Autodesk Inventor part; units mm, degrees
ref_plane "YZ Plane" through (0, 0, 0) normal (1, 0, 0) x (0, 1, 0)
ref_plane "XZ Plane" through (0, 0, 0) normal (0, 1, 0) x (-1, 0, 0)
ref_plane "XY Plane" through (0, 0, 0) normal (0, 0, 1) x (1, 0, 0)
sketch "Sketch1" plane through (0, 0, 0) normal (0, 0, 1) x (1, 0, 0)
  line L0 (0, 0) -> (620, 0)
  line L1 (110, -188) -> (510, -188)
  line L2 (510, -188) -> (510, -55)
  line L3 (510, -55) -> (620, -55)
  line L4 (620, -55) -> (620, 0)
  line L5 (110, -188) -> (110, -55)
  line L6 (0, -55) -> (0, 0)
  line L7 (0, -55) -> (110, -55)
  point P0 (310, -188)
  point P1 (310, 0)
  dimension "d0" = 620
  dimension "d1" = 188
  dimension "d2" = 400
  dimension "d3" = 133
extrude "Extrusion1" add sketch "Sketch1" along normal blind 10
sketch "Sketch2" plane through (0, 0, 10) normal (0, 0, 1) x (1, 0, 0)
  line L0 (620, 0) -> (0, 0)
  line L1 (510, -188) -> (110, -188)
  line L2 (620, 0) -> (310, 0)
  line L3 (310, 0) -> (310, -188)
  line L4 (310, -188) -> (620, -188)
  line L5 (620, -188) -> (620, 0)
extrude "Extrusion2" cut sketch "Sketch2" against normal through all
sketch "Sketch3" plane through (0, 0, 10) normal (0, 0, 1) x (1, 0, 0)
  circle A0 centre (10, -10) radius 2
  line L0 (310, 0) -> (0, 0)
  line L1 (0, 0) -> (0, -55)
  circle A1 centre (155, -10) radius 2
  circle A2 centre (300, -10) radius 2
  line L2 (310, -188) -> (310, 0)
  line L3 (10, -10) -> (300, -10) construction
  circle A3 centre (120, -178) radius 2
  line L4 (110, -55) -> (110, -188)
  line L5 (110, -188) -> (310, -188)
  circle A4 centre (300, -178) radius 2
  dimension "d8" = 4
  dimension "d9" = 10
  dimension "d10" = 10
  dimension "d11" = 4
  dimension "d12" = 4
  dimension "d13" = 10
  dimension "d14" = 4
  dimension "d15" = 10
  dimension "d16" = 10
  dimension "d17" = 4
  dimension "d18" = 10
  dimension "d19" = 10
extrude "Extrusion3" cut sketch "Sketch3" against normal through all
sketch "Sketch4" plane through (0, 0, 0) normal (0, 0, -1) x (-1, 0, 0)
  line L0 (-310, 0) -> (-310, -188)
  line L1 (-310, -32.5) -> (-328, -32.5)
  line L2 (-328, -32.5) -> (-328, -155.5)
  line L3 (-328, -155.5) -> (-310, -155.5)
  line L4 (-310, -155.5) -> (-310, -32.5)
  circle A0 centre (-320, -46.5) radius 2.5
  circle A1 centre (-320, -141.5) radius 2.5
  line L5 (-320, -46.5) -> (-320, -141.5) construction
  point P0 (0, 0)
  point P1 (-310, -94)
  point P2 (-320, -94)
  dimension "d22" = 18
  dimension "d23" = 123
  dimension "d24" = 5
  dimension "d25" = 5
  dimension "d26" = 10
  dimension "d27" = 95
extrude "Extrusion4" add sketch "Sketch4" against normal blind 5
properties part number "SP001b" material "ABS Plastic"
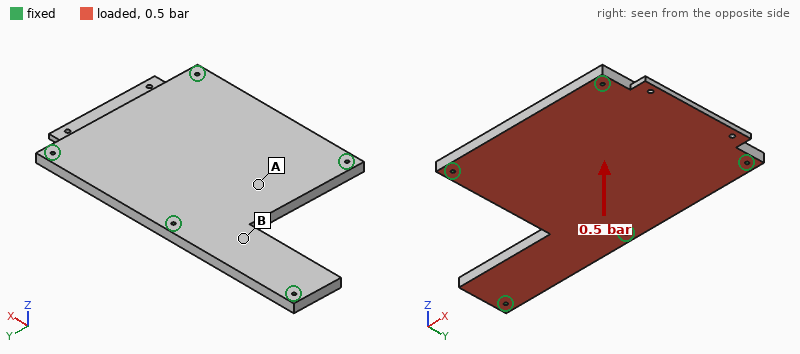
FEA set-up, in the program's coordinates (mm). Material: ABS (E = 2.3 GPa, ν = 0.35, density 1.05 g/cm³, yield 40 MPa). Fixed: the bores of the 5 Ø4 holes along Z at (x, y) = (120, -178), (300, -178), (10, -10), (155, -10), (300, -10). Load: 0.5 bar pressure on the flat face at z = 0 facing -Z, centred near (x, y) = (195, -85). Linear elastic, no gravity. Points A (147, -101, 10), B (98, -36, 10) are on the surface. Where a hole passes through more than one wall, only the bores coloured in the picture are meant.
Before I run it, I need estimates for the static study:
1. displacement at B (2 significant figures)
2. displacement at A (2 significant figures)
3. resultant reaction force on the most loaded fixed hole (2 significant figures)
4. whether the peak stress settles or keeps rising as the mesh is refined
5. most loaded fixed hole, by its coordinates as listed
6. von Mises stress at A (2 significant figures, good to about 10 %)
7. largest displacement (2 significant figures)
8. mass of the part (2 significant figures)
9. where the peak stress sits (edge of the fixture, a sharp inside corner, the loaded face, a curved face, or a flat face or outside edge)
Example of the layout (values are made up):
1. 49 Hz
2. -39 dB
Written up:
1. 0.73 mm
2. 1.4 mm
3. 680 N
4. keeps rising
5. (155, -10)
6. 5.7 MPa
7. 1.8 mm
8. 470 g
9. edge of the fixture
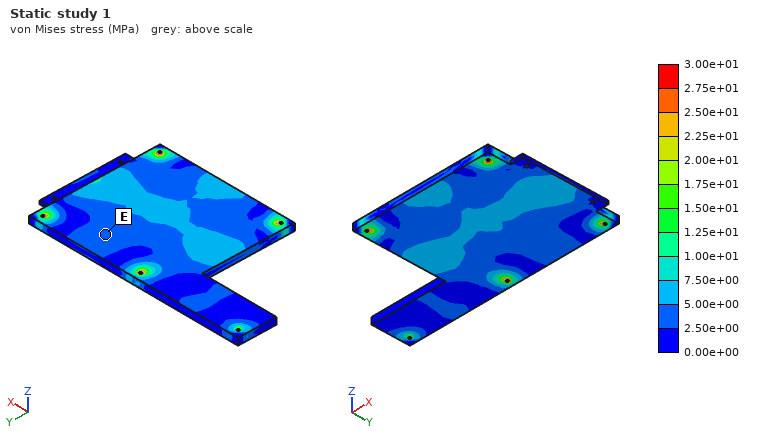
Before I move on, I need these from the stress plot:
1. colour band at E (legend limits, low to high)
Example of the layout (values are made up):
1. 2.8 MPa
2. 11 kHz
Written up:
1. 2.50e+00 to 5.00e+00 MPa
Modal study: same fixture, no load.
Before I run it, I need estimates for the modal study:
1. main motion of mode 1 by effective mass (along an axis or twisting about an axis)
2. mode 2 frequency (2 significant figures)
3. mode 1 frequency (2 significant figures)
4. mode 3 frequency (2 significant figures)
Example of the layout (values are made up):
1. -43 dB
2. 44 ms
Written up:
1. along Z
2. 450 Hz
3. 310 Hz
4. 480 Hz
